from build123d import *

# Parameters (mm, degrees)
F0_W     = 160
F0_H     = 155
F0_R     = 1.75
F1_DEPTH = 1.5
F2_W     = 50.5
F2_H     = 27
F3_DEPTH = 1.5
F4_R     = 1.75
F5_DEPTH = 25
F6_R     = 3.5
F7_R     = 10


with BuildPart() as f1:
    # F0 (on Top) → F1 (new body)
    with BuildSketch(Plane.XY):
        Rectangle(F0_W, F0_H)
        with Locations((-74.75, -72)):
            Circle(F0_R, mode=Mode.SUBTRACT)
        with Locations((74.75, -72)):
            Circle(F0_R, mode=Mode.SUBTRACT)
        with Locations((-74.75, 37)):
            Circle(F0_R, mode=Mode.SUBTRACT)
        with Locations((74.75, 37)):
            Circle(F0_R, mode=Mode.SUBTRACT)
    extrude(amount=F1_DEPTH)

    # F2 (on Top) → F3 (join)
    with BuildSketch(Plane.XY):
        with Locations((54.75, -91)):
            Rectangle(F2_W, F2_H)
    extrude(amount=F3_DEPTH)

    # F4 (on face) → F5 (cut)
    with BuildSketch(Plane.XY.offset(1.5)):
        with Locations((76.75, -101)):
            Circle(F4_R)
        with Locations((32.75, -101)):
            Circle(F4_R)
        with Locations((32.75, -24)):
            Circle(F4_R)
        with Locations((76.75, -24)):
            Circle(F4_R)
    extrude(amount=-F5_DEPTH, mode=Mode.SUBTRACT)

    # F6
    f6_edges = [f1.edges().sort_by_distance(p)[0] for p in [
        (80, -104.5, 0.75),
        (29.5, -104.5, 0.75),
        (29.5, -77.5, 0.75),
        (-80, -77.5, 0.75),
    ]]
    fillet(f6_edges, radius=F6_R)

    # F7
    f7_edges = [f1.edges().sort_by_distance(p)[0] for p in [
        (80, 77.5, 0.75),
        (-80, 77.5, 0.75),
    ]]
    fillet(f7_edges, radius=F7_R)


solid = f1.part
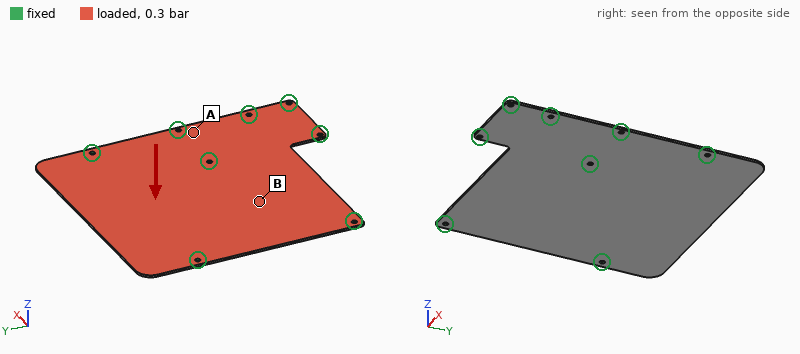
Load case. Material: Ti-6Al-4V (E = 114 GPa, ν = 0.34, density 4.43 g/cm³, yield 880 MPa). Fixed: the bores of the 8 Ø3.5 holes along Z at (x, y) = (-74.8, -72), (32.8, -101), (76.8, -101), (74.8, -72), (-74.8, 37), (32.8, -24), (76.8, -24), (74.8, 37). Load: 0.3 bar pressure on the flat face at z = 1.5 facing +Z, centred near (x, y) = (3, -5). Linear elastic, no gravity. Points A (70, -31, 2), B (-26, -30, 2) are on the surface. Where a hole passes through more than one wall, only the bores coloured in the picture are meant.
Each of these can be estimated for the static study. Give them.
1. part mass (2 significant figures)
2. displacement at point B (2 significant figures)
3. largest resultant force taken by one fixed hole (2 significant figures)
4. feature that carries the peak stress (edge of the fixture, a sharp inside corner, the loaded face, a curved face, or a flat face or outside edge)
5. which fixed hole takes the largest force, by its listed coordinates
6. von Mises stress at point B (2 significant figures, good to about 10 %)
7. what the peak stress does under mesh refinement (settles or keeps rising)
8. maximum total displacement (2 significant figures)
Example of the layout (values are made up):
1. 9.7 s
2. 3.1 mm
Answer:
1. 170 g
2. 0.67 mm
3. 250 N
4. edge of the fixture
5. (32.8, -24)
6. 45 MPa
7. keeps rising
8. 2.2 mm
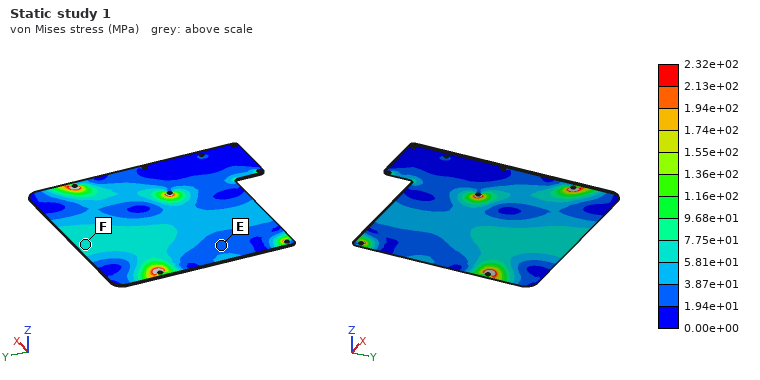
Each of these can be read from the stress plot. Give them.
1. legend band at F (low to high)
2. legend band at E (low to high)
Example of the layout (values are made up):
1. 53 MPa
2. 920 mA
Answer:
1. 5.81e+01 to 7.75e+01 MPa
2. 1.94e+01 to 3.87e+01 MPa
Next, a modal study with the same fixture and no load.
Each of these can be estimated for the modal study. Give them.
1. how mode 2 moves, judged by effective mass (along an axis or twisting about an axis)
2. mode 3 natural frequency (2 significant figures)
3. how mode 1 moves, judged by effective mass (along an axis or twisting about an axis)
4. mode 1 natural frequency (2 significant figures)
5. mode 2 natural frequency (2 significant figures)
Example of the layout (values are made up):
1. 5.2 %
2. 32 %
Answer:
1. along Z
2. 660 Hz
3. along Z
4. 300 Hz
5. 490 Hz
